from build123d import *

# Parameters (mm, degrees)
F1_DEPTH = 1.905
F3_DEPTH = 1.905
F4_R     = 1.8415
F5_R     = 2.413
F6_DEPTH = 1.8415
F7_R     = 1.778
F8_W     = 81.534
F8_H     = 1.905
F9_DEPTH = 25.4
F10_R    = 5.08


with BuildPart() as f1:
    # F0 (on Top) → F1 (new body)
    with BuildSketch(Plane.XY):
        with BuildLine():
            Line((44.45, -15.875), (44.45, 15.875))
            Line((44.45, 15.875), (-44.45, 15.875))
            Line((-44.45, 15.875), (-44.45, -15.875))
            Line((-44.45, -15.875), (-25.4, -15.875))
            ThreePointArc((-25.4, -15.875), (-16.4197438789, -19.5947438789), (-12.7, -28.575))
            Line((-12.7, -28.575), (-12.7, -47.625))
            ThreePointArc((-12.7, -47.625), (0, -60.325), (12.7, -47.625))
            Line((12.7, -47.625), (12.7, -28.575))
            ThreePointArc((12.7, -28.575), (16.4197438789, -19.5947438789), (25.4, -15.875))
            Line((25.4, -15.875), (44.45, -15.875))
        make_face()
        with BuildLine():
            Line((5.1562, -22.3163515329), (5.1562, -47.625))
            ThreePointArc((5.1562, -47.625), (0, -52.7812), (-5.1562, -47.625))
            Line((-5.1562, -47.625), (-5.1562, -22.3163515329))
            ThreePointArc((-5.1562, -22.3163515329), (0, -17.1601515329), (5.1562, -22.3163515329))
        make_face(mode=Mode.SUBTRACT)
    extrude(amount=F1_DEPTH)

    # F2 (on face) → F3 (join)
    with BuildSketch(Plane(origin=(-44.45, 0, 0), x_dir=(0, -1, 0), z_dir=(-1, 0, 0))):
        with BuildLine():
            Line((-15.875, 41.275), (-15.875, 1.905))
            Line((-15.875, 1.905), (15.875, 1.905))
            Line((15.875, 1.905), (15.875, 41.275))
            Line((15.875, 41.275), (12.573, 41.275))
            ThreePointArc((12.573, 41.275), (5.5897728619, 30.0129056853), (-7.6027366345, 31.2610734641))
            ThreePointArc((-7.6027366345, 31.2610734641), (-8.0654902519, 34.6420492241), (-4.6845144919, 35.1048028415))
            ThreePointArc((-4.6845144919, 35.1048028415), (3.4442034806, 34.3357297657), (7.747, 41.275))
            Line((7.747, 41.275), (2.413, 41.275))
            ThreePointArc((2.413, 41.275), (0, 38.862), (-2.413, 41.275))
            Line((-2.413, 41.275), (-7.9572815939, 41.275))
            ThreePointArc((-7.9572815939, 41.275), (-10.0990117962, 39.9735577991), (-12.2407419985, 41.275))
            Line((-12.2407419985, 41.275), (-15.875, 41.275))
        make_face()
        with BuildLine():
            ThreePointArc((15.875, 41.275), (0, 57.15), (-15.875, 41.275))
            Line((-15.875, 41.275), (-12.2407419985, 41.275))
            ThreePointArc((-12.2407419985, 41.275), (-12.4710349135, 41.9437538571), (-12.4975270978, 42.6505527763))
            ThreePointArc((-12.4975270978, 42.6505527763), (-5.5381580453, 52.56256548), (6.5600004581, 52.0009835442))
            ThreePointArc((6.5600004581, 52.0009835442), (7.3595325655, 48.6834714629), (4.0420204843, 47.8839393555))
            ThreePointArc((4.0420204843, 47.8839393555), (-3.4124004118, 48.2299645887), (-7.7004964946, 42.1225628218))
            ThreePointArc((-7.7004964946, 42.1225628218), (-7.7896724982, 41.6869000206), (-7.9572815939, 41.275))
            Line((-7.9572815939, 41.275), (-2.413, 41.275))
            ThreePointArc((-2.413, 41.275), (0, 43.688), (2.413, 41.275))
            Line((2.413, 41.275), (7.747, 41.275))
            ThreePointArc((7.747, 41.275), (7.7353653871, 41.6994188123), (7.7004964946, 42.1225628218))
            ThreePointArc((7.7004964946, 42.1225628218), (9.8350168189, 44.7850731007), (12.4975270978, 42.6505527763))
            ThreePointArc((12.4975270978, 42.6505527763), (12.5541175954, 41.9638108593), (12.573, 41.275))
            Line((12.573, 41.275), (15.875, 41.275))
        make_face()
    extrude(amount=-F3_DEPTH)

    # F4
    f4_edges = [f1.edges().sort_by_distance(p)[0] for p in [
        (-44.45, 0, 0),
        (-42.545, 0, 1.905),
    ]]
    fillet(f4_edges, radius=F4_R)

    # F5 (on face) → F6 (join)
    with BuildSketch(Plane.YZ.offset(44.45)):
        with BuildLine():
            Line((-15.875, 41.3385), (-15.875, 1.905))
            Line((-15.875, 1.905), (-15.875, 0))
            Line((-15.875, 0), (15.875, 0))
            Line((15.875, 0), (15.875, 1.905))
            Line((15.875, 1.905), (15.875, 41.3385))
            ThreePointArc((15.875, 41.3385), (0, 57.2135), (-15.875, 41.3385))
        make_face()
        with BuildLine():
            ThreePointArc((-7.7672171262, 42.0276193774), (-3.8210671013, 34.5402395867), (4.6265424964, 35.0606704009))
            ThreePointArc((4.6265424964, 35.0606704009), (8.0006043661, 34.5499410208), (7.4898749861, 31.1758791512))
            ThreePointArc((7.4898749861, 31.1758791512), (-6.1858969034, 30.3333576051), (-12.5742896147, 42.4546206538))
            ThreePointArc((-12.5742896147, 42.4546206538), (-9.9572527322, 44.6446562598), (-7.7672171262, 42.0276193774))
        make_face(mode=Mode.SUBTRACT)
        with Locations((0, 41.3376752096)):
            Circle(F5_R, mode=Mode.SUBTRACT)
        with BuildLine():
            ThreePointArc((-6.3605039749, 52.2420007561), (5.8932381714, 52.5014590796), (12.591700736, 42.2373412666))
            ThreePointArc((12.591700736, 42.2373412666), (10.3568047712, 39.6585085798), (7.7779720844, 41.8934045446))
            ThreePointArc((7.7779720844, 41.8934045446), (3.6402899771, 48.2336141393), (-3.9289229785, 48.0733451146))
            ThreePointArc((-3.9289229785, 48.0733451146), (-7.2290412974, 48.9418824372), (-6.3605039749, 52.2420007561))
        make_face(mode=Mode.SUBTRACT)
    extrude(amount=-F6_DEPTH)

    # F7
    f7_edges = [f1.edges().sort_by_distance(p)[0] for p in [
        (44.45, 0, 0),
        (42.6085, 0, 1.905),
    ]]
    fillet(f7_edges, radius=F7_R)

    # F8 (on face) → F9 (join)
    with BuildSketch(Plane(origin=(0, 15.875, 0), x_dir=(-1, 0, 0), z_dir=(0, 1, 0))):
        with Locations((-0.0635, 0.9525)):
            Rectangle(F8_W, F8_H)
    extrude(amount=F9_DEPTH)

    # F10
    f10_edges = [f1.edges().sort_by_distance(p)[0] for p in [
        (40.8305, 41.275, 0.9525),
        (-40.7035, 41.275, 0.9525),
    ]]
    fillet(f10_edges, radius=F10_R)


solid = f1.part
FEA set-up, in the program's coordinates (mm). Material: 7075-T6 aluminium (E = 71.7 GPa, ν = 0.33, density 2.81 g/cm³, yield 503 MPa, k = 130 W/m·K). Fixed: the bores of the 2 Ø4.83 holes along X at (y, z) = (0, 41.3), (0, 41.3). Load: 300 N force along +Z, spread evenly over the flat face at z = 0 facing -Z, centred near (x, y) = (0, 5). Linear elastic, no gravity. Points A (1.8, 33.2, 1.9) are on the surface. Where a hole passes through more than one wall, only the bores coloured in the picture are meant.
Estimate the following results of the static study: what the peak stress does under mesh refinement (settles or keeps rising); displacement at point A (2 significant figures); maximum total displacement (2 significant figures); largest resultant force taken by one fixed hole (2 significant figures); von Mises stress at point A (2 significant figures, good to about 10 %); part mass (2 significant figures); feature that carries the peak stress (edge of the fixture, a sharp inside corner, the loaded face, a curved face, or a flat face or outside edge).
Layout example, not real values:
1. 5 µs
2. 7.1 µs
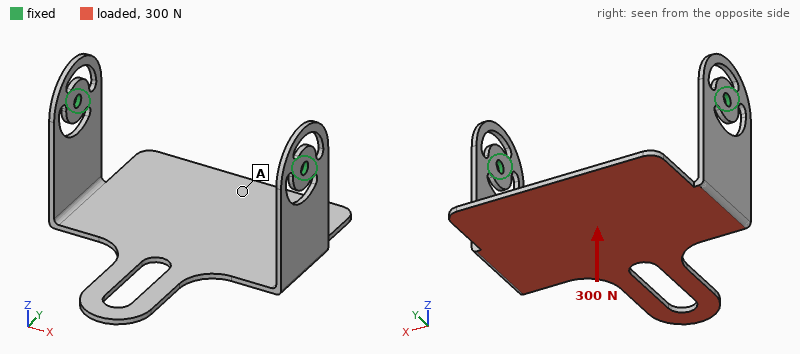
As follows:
1. keeps rising
2. 0.74 mm
3. 1.7 mm
4. 160 N
5. 50 MPa
6. 45 g
7. a sharp inside corner
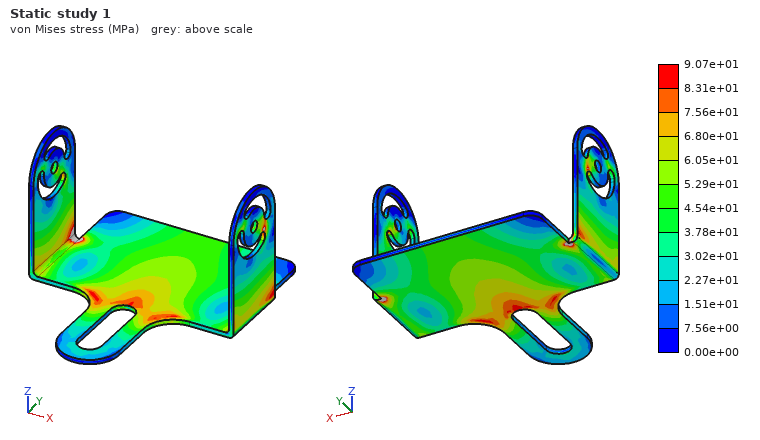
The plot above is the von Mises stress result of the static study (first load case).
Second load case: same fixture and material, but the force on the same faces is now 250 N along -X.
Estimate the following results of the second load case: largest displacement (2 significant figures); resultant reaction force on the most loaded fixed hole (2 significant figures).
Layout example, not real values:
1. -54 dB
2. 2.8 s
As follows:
1. 1.6 mm
2. 150 N
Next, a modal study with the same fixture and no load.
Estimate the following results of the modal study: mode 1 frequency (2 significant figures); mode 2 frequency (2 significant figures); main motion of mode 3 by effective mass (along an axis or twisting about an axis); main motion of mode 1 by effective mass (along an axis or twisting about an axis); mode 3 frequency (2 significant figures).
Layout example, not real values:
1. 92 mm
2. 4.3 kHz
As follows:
1. 330 Hz
2. 490 Hz
3. along Z
4. along X
5. 680 Hz
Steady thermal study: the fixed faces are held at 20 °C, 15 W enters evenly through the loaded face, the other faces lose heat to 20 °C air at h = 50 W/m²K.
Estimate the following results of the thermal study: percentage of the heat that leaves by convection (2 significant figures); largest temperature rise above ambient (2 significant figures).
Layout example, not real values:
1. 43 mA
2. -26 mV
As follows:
1. 80 %
2. 30 K
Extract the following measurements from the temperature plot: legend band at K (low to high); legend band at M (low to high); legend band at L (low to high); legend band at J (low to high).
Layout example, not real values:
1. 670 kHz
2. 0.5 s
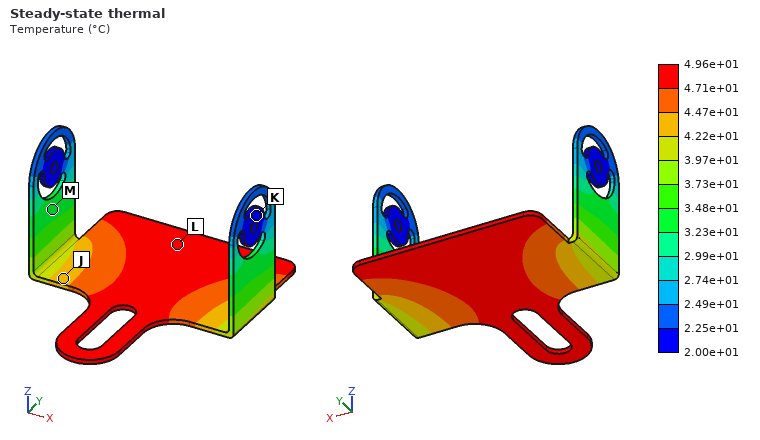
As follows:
1. 2.00e+01 to 2.25e+01 °C
2. 3.23e+01 to 3.48e+01 °C
3. 4.71e+01 to 4.96e+01 °C
4. 4.22e+01 to 4.47e+01 °C
